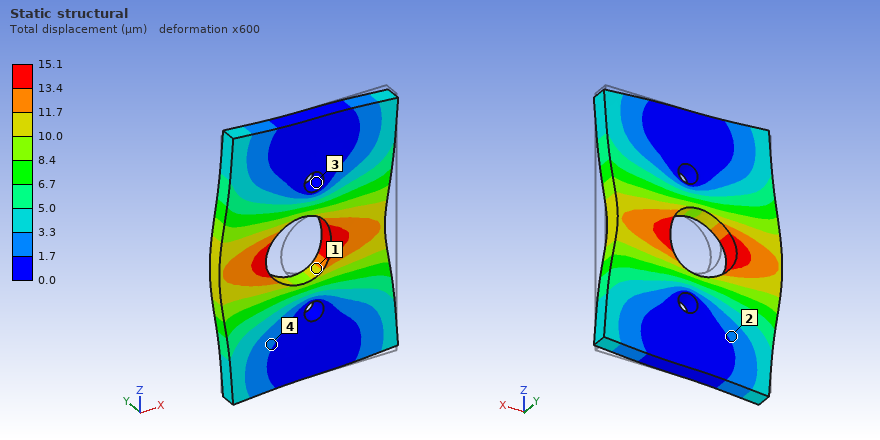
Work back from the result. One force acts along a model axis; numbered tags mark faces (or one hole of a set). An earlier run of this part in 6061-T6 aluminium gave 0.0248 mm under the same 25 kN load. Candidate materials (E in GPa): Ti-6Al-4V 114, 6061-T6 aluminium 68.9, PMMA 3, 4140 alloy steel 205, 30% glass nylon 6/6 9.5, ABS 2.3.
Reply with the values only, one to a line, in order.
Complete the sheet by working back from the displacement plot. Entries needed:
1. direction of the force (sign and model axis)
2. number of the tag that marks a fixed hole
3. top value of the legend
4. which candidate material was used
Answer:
-X
3
15.1 µm
Ti-6Al-4V
